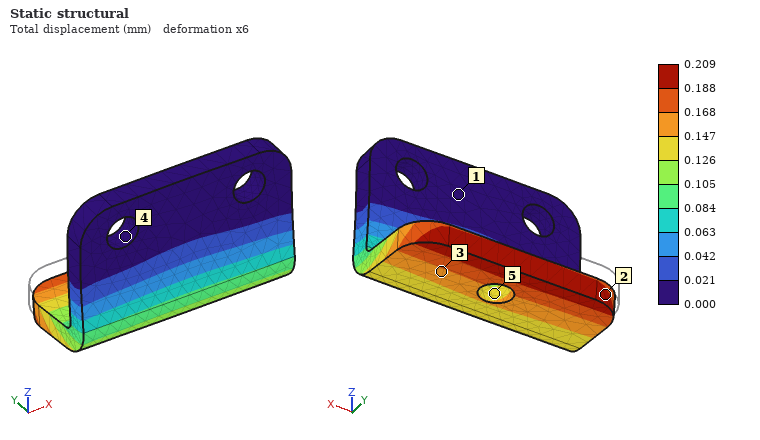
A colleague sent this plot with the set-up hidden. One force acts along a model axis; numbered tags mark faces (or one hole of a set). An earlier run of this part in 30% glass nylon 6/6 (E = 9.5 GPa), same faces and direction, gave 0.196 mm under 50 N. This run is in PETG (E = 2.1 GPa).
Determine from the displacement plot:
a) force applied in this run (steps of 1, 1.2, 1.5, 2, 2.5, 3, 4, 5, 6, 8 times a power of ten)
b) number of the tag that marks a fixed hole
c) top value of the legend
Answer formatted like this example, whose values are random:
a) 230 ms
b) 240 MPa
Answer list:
a) 12 N
b) 4
c) 0.209 mm
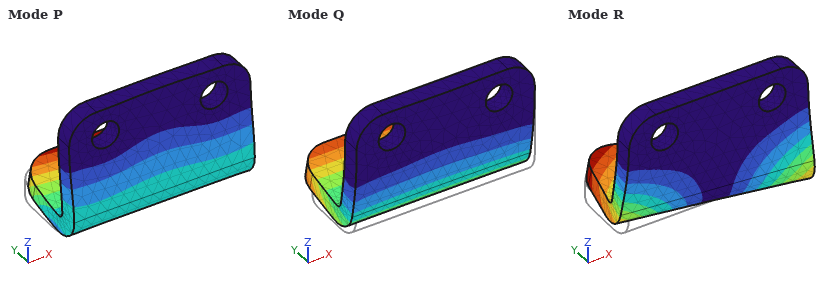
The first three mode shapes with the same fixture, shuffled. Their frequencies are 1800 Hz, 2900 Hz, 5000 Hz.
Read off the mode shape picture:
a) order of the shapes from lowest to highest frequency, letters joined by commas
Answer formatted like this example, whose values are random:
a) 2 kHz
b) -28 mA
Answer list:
a) Q, R, P
